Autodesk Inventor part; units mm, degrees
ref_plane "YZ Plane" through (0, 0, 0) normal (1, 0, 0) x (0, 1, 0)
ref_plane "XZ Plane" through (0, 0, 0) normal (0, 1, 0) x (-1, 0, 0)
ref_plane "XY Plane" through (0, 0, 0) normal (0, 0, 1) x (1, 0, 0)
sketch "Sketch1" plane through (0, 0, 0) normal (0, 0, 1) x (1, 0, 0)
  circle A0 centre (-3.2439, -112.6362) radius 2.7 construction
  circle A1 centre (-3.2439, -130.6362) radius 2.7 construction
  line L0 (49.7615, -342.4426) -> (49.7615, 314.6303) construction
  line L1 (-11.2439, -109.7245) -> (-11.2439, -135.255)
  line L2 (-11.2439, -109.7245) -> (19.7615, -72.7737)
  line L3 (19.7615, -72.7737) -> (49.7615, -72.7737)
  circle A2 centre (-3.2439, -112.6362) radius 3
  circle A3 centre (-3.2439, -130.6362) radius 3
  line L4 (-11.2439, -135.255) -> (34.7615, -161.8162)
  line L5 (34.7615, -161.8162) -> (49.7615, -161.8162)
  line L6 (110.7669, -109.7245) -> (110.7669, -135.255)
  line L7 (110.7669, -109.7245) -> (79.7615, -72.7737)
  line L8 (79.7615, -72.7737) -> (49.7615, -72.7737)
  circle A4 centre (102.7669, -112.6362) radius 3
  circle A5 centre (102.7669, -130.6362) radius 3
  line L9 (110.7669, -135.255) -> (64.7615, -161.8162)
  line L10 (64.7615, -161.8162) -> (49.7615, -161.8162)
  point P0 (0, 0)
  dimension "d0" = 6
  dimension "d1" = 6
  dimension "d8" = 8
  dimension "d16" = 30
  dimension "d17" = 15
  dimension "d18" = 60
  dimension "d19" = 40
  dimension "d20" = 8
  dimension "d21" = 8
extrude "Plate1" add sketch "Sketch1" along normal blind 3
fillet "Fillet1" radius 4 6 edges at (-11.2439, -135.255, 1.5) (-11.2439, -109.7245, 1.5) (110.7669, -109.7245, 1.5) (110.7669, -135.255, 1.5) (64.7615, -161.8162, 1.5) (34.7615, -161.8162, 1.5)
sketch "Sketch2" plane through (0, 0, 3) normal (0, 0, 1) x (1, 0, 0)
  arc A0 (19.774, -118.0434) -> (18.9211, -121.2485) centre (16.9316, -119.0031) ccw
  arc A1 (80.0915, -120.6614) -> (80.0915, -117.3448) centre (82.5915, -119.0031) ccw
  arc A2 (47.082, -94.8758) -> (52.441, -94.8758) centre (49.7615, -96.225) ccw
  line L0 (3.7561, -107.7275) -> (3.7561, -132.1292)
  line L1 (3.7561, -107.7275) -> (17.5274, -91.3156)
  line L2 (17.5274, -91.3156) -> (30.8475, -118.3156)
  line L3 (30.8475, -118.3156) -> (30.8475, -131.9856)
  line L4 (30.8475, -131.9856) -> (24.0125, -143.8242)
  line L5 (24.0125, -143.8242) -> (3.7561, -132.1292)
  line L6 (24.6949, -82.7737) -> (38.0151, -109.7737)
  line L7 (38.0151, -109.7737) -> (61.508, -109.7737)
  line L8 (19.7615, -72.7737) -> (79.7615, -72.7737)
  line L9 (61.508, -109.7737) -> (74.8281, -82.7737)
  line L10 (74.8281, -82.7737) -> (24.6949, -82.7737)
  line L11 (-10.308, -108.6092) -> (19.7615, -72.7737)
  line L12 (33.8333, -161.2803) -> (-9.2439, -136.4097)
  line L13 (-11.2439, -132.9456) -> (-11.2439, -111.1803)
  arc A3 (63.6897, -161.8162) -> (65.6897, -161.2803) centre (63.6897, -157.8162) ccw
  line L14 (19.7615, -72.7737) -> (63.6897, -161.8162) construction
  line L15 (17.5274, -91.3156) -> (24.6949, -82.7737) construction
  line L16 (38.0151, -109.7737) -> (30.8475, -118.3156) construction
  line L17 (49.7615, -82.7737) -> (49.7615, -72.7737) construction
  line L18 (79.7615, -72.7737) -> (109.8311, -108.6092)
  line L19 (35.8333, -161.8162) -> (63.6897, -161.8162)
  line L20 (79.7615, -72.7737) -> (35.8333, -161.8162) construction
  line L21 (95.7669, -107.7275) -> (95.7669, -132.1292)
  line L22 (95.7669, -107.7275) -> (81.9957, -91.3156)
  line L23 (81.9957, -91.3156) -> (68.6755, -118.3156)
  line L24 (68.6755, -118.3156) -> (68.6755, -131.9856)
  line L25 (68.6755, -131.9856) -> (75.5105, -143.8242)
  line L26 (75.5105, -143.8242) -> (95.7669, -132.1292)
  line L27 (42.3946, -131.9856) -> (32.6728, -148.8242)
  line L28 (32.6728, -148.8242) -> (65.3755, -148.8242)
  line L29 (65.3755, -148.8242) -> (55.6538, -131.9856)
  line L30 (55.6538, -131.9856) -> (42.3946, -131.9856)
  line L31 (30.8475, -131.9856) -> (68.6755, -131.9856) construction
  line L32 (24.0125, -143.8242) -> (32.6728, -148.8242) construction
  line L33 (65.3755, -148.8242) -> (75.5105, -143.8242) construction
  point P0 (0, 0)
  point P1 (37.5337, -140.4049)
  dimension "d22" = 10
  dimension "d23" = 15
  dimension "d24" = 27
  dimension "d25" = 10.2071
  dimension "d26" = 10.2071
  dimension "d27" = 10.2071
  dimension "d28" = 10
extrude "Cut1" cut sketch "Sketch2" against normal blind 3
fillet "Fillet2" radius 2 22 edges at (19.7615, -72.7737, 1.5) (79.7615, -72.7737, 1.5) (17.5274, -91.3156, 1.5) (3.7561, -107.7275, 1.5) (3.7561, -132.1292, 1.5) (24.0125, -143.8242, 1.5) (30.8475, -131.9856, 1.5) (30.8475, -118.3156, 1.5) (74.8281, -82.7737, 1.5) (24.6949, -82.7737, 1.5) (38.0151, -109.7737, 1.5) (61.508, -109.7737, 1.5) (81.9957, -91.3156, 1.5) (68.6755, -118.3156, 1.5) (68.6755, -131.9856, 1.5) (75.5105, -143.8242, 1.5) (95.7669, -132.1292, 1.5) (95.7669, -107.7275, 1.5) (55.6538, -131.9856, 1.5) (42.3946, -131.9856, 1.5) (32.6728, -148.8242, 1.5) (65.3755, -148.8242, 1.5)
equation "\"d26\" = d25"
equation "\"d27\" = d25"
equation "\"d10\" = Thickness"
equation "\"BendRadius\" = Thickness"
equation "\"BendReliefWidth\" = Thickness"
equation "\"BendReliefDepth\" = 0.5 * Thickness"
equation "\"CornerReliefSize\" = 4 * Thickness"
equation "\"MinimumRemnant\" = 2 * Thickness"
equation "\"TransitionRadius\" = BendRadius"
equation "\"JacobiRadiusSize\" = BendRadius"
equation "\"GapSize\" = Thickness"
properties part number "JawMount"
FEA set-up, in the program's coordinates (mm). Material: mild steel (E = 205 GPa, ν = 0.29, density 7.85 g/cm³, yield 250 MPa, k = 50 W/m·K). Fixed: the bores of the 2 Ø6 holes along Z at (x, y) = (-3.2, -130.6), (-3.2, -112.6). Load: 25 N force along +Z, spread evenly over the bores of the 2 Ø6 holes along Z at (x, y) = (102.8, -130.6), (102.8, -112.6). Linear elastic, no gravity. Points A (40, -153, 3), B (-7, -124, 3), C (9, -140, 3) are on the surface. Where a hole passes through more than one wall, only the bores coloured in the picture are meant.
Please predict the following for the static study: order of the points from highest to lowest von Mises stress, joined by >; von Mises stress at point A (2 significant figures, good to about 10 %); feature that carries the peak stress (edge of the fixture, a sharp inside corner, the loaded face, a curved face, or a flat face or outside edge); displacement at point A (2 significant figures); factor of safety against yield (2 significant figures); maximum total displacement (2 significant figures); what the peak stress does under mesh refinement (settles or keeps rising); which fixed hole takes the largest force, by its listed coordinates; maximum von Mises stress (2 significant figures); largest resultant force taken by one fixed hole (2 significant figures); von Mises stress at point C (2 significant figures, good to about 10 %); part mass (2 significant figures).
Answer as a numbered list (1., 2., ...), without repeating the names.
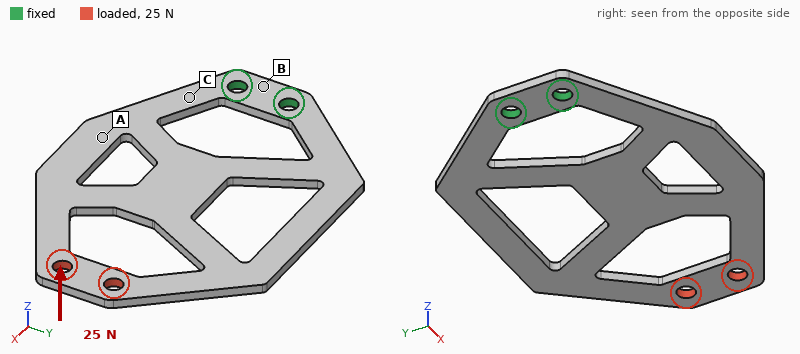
1. C > A > B
2. 26 MPa
3. a curved face
4. 0.23 mm
5. 2.1
6. 1.0 mm
7. settles
8. (-3.2, -130.6)
9. 120 MPa
10. 19 N
11. 83 MPa
12. 120 g
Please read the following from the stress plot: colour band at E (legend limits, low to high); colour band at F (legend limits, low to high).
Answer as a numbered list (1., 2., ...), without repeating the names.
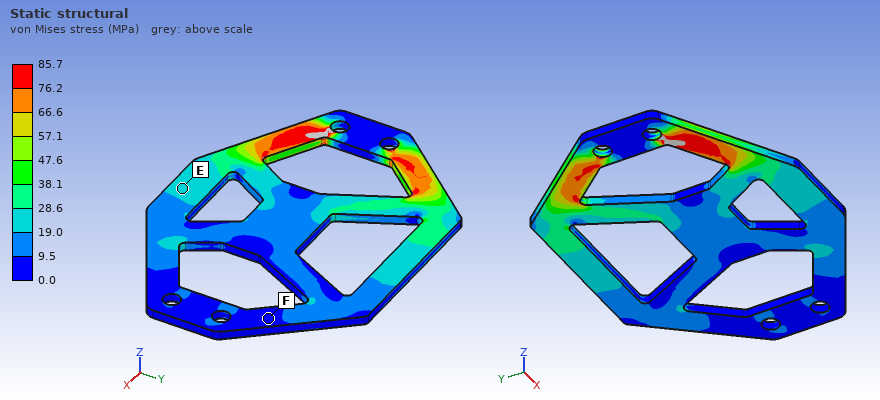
1. 19.0 to 28.6 MPa
2. 0.0 to 9.5 MPa
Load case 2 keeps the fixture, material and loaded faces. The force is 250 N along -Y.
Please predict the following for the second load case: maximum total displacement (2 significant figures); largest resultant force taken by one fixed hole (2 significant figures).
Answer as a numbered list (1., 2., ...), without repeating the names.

1. 0.13 mm
2. 760 N
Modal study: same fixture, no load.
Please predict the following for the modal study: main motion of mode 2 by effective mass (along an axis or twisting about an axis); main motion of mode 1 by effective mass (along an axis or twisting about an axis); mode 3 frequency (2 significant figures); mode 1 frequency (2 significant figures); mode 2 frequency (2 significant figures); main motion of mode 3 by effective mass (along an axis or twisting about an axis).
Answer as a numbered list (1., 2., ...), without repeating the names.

1. twisting about X
2. along Z
3. 900 Hz
4. 150 Hz
5. 450 Hz
6. along Z
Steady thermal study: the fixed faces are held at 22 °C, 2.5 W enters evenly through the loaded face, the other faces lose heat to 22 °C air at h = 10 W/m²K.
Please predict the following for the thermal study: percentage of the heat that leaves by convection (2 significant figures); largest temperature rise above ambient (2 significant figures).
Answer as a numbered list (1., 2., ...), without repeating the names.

1. 72 %
2. 41 K
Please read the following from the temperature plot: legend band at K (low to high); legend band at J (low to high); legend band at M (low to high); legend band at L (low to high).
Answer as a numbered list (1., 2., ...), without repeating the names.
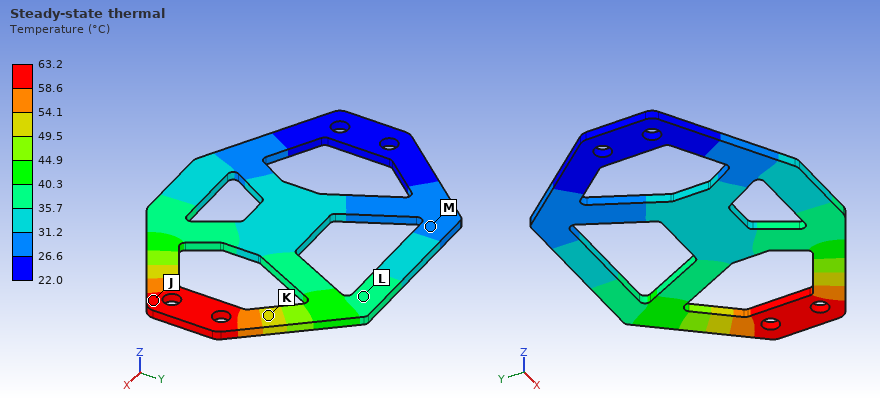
1. 49.5 to 54.1 °C
2. 58.6 to 63.2 °C
3. 26.6 to 31.2 °C
4. 35.7 to 40.3 °C
